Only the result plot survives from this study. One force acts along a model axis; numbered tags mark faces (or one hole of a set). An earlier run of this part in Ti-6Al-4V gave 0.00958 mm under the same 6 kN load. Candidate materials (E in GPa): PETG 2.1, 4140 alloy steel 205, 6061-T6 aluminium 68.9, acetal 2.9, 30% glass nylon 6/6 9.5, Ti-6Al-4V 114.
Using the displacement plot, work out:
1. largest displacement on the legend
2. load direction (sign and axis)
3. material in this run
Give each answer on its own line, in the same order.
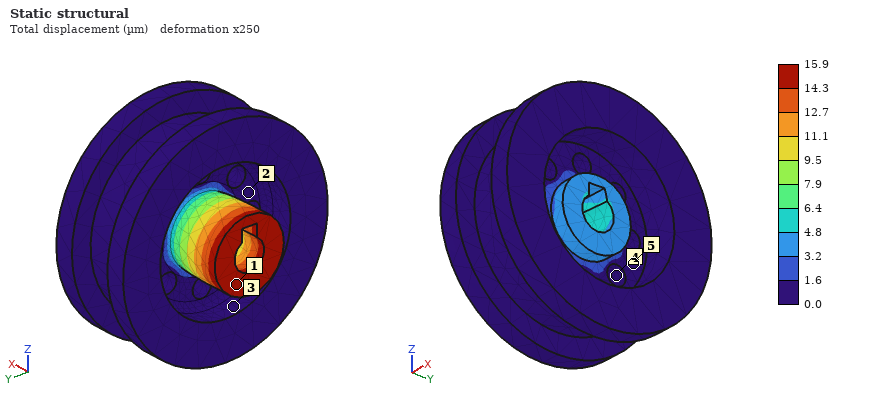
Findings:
15.9 µm
+X
6061-T6 aluminium
